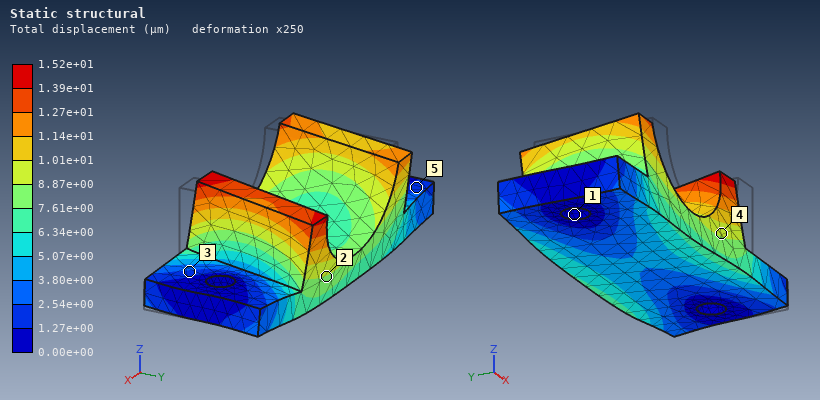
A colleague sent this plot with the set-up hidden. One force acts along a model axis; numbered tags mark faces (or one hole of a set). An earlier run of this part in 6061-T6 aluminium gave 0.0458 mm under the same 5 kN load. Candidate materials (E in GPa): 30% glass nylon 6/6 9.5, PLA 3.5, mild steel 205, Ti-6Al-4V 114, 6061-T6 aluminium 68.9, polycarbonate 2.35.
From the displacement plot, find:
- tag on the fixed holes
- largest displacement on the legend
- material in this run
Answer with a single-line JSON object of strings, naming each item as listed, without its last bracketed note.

{"tag on the fixed holes": "1", "largest displacement on the legend": "1.52e+01 µm", "material in this run": "mild steel"}
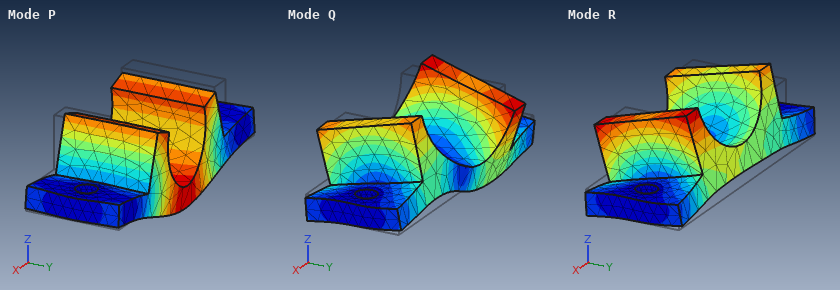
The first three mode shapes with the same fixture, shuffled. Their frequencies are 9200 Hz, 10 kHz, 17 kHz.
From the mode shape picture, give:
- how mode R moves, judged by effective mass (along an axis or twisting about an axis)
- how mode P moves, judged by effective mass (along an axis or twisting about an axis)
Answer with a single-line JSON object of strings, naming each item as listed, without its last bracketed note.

{"how mode R moves, judged by effective mass": "along Y", "how mode P moves, judged by effective mass": "along Z"}
